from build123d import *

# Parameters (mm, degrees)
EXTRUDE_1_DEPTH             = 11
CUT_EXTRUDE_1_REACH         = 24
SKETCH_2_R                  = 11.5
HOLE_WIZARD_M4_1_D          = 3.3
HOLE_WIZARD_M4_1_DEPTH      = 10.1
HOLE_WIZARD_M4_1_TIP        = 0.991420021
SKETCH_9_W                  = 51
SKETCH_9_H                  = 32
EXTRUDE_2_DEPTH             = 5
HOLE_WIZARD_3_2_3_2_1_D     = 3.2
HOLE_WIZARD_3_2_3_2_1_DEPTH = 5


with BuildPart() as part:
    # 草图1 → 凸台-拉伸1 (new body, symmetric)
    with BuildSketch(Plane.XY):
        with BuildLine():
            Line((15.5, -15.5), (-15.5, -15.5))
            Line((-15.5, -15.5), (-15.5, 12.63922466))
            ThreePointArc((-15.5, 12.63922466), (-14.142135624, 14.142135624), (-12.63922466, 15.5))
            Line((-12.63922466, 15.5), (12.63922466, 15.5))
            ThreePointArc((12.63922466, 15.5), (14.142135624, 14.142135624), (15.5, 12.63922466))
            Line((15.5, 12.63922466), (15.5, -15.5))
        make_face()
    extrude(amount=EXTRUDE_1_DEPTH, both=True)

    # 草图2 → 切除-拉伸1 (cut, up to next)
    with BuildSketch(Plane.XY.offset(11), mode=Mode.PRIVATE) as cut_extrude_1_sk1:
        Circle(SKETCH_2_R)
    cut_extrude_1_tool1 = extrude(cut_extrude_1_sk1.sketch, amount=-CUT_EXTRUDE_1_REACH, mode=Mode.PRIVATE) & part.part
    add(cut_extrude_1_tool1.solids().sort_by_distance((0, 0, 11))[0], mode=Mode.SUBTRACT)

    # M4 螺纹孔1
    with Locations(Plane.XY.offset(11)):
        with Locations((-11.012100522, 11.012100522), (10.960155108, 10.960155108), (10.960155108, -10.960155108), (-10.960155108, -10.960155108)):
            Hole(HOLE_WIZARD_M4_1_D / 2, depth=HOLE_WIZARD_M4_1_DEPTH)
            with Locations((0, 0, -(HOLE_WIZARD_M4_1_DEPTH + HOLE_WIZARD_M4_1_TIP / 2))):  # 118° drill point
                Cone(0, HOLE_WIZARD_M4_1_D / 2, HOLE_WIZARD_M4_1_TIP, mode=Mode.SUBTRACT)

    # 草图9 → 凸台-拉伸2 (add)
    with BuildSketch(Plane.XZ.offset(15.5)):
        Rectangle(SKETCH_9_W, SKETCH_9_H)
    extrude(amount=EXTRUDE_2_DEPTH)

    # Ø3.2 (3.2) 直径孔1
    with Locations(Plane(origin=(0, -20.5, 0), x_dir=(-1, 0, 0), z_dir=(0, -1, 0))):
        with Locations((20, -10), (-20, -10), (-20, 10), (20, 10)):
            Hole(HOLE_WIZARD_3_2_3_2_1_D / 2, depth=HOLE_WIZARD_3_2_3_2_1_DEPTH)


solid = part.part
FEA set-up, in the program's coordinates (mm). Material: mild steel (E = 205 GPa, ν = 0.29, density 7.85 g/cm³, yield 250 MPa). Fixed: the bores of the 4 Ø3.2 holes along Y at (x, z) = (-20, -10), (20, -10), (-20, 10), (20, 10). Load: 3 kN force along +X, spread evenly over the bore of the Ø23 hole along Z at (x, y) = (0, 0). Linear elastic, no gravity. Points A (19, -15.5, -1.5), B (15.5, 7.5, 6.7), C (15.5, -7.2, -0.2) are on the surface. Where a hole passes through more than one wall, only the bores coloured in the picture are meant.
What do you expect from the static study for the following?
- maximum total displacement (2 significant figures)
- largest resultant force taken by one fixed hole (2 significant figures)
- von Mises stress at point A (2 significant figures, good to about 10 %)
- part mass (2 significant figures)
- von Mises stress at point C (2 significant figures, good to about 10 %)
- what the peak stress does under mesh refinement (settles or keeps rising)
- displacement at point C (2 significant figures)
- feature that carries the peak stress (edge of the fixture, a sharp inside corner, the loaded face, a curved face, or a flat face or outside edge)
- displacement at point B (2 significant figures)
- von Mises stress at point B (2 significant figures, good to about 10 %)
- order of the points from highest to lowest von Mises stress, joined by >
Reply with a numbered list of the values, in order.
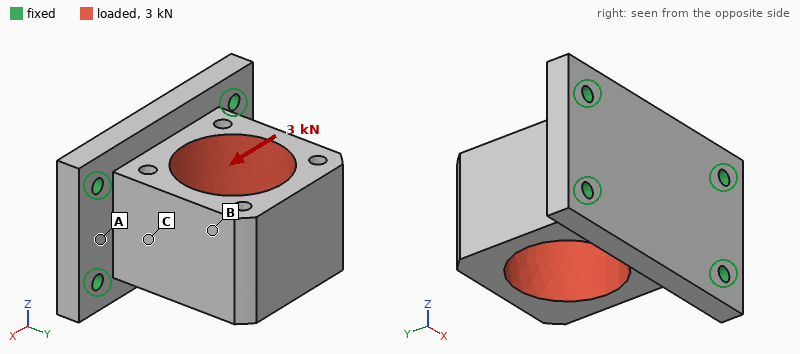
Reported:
1. 19 µm
2. 1.1 kN
3. 13 MPa
4. 150 g
5. 43 MPa
6. keeps rising
7. 5.2 µm
8. edge of the fixture
9. 16 µm
10. 28 MPa
11. C > B > A
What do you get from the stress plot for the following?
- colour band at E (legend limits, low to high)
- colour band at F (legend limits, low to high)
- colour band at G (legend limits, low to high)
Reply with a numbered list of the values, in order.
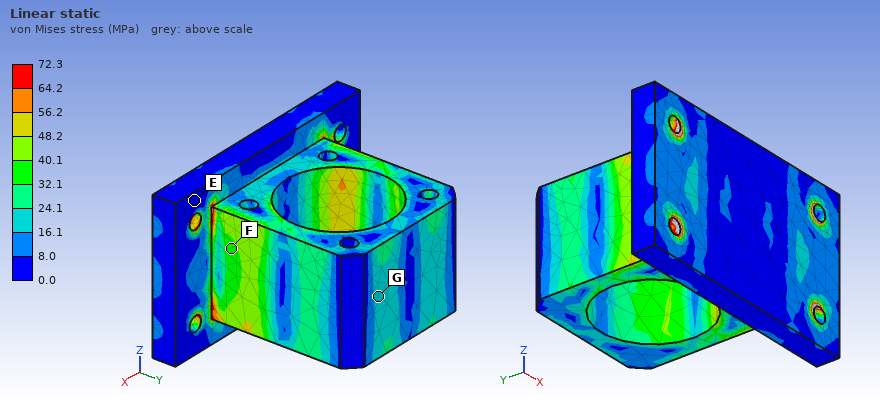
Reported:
1. 0.0 to 8.0 MPa
2. 32.1 to 40.1 MPa
3. 16.1 to 24.1 MPa
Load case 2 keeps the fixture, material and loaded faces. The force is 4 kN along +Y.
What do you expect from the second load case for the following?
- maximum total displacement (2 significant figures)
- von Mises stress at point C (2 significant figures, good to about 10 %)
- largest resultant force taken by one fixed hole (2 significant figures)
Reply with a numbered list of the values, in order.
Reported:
1. 6.6 µm
2. 22 MPa
3. 1.1 kN
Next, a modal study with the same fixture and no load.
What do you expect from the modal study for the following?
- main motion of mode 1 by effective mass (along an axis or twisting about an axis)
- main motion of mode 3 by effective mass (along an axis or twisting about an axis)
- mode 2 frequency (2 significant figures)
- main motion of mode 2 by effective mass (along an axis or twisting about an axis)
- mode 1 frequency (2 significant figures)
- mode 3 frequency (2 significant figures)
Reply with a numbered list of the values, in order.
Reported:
1. along Z
2. twisting about Y
3. 7400 Hz
4. along X
5. 6700 Hz
6. 13 kHz
